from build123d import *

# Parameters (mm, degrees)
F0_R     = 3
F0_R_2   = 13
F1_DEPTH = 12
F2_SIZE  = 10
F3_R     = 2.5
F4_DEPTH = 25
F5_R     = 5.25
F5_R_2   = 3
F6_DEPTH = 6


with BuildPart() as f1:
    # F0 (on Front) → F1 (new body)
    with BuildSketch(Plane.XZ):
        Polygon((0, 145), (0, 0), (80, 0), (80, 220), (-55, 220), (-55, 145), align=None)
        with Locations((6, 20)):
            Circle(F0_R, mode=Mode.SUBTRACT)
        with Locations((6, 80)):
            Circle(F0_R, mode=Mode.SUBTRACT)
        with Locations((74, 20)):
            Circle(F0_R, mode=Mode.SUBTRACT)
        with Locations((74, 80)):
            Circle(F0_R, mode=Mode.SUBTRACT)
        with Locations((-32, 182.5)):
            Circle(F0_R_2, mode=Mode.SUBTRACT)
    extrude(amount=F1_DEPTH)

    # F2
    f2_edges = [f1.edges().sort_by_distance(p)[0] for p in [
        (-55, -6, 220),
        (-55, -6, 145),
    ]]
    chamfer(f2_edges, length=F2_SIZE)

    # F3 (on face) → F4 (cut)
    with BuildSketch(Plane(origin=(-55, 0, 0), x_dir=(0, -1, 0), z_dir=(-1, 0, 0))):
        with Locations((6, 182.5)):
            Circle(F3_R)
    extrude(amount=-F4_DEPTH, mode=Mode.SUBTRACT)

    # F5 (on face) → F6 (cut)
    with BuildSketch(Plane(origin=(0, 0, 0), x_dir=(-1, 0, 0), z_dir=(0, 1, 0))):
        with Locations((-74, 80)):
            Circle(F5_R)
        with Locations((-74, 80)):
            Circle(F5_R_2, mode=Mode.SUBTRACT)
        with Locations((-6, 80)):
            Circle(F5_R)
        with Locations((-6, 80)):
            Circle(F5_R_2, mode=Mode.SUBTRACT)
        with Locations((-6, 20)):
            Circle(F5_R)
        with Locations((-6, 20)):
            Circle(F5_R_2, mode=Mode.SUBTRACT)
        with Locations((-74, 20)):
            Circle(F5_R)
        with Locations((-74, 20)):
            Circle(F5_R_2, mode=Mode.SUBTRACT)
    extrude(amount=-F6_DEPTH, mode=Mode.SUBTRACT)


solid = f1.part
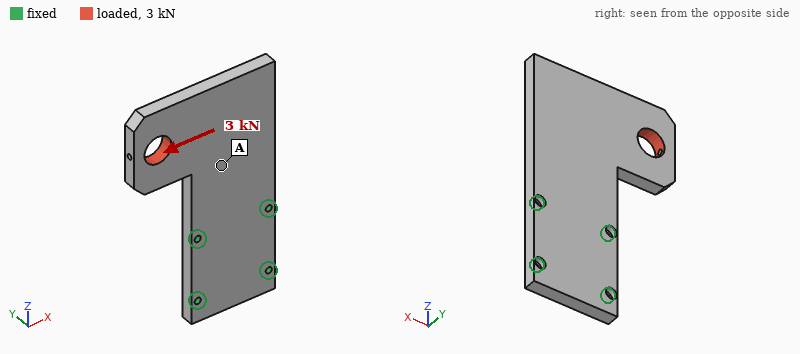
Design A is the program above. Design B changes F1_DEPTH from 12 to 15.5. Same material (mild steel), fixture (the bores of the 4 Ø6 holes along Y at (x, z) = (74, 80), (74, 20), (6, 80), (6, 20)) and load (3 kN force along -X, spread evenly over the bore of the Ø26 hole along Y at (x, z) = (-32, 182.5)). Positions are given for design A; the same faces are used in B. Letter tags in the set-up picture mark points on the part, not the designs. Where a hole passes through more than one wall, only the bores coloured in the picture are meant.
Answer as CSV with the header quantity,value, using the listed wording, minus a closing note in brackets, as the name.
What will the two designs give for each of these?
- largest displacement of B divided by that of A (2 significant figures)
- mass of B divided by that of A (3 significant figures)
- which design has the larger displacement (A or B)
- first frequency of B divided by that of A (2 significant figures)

quantity,value
largest displacement of B divided by that of A,0.72
mass of B divided by that of A,1.29
which design has the larger displacement,A
first frequency of B divided by that of A,1.3
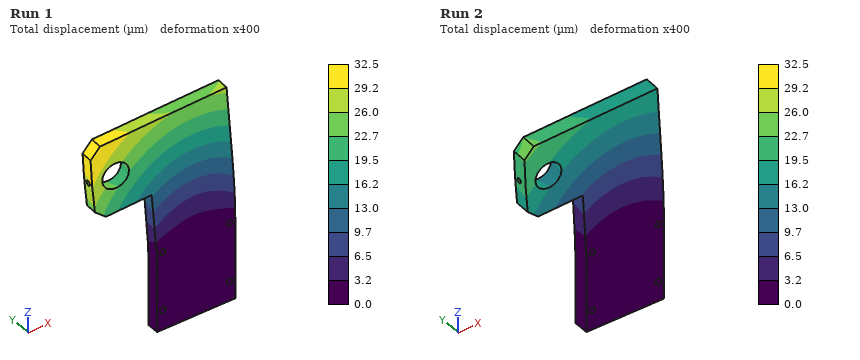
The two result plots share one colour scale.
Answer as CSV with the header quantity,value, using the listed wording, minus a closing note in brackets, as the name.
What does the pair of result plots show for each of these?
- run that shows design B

quantity,value
run that shows design B,Run 2
